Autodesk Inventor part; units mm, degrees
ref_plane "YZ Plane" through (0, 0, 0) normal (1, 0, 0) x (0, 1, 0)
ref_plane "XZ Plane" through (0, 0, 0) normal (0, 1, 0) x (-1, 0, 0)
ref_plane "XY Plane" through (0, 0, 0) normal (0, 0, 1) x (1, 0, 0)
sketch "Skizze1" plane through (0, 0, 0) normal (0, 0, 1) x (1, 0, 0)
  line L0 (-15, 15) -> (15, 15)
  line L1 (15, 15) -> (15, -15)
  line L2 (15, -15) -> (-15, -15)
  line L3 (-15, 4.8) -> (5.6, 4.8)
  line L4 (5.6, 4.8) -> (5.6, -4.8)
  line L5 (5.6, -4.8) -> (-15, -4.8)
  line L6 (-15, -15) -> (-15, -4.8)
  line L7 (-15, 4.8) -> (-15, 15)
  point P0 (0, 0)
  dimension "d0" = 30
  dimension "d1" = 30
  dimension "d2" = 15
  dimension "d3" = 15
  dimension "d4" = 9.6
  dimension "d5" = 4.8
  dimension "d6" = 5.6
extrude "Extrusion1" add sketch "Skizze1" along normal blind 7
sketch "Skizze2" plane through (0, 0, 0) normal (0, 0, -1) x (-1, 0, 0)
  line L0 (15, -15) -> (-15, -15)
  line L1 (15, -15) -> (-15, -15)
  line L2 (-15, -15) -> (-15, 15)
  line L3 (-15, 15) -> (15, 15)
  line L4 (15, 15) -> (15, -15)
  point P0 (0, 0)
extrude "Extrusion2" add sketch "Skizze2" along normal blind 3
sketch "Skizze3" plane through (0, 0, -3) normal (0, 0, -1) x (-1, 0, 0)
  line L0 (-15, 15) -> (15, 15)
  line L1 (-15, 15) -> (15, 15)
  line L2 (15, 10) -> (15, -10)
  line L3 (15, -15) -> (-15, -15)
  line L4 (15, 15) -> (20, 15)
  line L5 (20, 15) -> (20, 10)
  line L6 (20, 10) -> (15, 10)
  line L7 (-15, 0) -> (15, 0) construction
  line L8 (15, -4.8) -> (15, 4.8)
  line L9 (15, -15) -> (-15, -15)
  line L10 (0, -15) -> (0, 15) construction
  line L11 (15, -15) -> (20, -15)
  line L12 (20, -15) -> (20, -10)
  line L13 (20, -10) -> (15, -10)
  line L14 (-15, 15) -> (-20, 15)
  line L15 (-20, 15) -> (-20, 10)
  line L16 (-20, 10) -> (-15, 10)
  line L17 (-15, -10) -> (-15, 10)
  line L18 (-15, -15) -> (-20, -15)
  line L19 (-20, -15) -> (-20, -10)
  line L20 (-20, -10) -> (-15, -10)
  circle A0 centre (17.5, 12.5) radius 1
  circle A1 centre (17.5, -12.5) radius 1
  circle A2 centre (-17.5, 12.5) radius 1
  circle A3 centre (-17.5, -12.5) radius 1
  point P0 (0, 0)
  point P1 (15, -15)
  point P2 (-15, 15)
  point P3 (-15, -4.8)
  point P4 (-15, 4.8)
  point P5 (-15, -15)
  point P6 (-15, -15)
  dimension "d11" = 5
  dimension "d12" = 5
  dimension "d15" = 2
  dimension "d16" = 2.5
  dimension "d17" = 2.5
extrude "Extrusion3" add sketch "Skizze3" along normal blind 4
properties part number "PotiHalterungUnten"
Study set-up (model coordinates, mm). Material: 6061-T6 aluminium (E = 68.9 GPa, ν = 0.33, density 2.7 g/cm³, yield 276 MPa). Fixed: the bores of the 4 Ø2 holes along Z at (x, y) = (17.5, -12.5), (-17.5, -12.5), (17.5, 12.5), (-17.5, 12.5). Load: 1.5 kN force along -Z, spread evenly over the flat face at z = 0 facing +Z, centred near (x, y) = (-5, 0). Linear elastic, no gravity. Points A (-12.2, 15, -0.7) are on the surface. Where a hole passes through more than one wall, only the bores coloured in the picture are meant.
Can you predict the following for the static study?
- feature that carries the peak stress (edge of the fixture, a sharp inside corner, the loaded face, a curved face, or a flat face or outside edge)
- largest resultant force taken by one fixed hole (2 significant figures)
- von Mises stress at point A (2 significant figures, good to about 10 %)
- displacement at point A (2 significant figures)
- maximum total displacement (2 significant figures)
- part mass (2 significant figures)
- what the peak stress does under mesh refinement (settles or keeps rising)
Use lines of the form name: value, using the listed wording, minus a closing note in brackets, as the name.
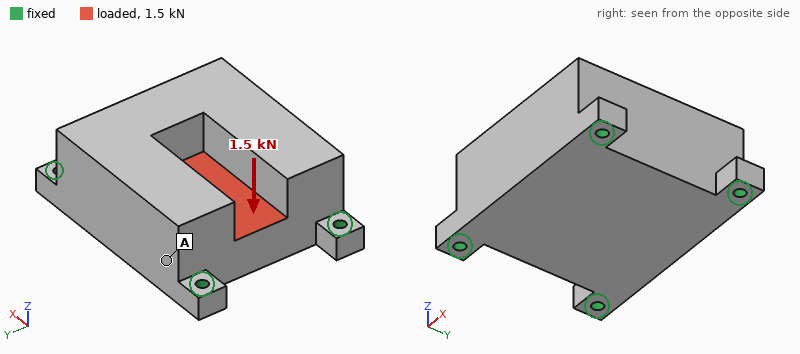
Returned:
feature that carries the peak stress: edge of the fixture
largest resultant force taken by one fixed hole: 530 N
von Mises stress at point A: 17 MPa
displacement at point A: 3.9 µm
maximum total displacement: 12 µm
part mass: 31 g
what the peak stress does under mesh refinement: keeps rising
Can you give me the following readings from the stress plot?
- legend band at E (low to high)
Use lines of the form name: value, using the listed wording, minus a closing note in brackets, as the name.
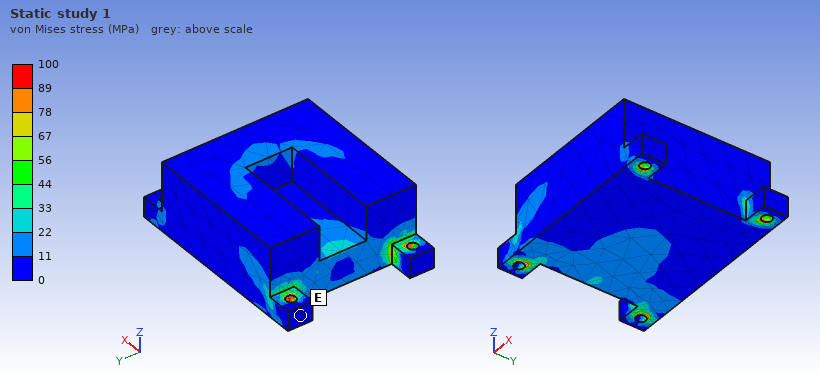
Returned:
legend band at E: 0 to 11 MPa
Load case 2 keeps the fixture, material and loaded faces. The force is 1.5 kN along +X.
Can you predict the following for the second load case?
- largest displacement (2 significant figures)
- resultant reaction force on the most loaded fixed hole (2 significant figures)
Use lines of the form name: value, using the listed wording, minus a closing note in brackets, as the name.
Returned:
largest displacement: 5.4 µm
resultant reaction force on the most loaded fixed hole: 410 N
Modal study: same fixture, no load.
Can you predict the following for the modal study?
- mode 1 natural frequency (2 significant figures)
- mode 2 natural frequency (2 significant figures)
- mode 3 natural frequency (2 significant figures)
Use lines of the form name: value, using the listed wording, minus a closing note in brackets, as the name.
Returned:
mode 1 natural frequency: 15 kHz
mode 2 natural frequency: 15 kHz
mode 3 natural frequency: 21 kHz
